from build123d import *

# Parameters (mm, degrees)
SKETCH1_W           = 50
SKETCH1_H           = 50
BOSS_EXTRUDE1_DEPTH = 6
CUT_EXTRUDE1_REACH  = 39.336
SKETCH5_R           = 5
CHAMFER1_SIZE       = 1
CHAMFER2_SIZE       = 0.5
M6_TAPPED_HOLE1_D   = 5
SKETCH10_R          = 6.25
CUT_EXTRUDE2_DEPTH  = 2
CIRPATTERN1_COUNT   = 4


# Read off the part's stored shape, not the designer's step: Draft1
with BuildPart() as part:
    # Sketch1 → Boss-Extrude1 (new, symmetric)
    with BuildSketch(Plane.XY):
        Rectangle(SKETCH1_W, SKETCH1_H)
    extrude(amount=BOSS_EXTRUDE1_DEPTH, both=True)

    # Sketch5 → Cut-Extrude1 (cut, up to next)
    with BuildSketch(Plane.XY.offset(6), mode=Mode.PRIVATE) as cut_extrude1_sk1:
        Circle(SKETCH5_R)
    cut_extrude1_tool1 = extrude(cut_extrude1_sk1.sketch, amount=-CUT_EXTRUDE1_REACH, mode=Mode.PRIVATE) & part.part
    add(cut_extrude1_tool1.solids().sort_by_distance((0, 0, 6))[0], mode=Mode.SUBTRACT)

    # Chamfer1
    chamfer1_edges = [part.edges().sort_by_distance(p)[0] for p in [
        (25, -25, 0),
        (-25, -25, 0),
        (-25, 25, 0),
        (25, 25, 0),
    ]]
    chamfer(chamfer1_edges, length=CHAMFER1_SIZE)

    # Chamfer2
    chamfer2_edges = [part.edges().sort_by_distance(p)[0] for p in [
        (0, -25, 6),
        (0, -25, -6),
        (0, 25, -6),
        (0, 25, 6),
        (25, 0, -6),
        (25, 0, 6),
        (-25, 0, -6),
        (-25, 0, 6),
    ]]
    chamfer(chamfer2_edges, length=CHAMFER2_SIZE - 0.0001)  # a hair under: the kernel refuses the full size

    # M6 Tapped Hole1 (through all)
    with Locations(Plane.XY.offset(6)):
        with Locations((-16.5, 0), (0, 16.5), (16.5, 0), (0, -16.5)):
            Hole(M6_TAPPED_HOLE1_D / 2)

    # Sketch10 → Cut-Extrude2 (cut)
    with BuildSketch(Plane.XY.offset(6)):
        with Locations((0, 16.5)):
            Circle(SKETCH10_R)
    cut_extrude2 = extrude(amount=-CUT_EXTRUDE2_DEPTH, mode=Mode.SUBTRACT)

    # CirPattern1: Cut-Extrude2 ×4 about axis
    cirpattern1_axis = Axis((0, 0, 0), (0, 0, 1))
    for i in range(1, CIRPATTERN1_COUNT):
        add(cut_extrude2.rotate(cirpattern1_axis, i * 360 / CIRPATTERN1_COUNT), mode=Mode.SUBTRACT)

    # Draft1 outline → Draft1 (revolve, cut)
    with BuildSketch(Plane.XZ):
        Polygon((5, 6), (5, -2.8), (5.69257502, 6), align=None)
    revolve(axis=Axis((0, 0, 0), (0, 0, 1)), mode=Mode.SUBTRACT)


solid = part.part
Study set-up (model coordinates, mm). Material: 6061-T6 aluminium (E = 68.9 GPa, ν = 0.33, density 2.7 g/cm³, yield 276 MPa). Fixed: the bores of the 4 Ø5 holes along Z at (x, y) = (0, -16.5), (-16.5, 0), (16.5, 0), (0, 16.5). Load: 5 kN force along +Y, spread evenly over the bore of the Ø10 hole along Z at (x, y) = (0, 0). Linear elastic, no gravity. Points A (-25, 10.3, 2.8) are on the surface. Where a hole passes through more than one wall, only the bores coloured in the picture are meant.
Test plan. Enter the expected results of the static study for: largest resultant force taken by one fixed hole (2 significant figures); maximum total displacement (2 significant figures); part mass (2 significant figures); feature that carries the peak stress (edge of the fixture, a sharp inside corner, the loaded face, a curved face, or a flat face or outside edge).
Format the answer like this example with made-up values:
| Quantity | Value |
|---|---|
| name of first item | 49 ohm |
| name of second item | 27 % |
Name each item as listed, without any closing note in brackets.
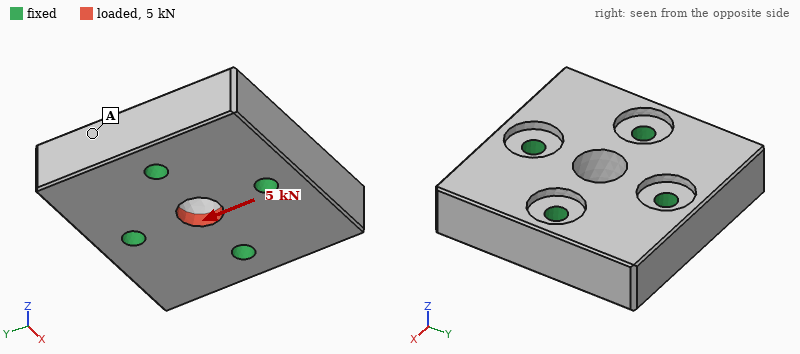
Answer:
| Quantity | Value |
|---|---|
| largest resultant force taken by one fixed hole | 1.7 kN |
| maximum total displacement | 5.8 µm |
| part mass | 73 g |
| feature that carries the peak stress | the loaded face |
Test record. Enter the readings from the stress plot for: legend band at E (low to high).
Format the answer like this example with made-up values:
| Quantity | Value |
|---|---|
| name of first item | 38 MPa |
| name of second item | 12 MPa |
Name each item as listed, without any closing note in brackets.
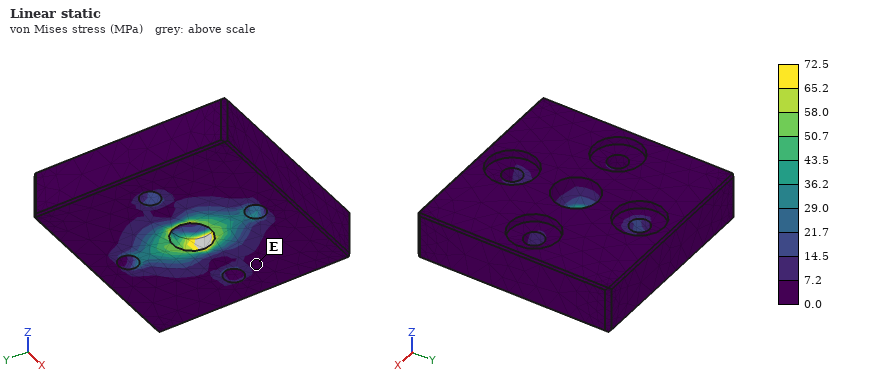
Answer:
| Quantity | Value |
|---|---|
| legend band at E | 0.0 to 7.2 MPa |
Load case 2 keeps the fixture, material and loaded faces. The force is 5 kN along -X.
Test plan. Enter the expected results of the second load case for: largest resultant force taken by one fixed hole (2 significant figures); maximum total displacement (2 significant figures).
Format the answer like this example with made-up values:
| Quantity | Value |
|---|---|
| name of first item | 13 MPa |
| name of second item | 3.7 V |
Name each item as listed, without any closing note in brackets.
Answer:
| Quantity | Value |
|---|---|
| largest resultant force taken by one fixed hole | 1.7 kN |
| maximum total displacement | 5.7 µm |
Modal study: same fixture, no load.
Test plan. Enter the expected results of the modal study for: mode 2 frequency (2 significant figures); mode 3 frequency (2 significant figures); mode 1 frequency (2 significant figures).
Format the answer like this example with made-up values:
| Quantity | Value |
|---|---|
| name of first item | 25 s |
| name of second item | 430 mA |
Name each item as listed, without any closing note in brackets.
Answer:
| Quantity | Value |
|---|---|
| mode 2 frequency | 20 kHz |
| mode 3 frequency | 20 kHz |
| mode 1 frequency | 19 kHz |
